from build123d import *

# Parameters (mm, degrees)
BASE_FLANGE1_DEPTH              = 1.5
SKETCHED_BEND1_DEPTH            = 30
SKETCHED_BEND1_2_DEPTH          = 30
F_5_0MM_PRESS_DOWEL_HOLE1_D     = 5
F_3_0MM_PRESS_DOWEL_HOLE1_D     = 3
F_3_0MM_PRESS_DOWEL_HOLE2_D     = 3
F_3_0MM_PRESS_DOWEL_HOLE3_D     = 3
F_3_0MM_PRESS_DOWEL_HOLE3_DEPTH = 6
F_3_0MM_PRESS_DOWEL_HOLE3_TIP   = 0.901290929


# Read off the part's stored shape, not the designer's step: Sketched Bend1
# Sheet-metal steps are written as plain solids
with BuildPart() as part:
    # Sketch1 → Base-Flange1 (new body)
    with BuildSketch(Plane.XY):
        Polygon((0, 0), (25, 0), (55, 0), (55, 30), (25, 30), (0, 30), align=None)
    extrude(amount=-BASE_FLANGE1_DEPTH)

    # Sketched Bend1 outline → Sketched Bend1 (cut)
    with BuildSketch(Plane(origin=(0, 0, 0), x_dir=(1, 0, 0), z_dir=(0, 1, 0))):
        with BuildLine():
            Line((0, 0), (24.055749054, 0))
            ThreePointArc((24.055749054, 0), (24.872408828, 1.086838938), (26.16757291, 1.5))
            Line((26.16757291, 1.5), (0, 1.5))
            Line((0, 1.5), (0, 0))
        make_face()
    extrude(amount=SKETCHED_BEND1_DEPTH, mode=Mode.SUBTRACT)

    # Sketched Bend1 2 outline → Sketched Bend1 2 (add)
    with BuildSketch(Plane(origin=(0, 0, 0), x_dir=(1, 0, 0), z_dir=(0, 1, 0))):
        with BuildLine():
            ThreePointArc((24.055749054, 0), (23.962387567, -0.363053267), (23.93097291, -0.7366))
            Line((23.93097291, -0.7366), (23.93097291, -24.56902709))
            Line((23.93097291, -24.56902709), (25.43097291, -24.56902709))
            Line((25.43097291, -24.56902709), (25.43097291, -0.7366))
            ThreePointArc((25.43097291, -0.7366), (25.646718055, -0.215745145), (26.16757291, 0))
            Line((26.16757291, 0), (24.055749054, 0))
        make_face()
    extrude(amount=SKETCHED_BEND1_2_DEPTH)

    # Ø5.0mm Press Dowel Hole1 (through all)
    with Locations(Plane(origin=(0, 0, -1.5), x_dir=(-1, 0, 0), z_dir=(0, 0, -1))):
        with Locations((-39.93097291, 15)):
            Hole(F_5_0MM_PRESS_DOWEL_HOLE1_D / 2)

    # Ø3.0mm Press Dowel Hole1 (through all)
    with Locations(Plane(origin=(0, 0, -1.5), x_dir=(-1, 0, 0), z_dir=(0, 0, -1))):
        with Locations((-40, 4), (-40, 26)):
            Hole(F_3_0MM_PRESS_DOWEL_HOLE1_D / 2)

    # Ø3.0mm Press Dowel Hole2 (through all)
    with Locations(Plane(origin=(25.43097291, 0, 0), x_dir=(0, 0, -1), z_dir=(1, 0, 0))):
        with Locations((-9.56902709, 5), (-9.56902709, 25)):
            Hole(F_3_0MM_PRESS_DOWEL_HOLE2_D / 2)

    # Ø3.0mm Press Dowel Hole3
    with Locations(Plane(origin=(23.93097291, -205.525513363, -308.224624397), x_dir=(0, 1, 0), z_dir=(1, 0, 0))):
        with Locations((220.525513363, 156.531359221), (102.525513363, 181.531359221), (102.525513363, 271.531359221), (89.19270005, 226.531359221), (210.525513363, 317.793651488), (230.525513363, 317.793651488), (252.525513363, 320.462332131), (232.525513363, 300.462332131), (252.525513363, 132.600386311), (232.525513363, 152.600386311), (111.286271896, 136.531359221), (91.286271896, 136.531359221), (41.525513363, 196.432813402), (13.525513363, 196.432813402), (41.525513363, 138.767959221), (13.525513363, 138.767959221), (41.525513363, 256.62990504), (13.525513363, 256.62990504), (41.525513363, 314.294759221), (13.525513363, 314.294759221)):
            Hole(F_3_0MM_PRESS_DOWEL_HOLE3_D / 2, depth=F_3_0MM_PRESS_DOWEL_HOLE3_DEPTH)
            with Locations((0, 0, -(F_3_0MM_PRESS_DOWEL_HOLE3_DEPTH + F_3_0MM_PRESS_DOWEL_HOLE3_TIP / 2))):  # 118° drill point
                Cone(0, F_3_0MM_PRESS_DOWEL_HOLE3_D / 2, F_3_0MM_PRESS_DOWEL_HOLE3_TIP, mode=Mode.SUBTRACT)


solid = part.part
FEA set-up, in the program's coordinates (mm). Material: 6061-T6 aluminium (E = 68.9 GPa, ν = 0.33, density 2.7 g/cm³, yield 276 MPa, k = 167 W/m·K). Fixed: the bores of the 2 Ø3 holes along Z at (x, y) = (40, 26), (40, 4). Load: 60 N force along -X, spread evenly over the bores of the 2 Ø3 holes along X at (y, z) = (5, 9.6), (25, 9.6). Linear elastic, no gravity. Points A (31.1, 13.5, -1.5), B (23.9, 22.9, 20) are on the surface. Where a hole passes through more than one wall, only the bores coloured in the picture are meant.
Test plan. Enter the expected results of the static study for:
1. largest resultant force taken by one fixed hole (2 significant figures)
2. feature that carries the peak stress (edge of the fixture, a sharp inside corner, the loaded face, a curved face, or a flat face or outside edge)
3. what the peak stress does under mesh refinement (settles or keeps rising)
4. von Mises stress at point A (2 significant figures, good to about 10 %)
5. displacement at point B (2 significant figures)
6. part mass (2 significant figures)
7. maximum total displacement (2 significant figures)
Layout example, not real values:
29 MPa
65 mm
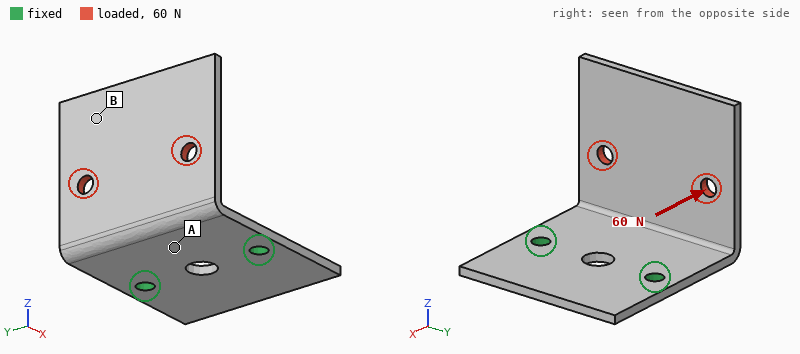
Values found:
31 N
edge of the fixture
keeps rising
45 MPa
0.42 mm
6.5 g
0.51 mm
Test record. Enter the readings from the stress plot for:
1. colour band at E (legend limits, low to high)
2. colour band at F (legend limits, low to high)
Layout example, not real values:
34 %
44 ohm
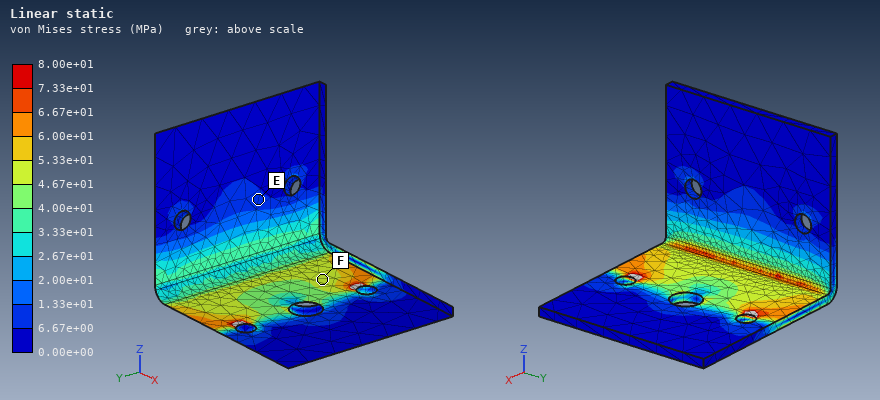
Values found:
6.67e+00 to 1.33e+01 MPa
4.67e+01 to 5.33e+01 MPa
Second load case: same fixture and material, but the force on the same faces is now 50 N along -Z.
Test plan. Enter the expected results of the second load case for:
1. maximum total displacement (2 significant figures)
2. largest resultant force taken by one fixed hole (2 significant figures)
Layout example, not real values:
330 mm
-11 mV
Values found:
0.27 mm
25 N
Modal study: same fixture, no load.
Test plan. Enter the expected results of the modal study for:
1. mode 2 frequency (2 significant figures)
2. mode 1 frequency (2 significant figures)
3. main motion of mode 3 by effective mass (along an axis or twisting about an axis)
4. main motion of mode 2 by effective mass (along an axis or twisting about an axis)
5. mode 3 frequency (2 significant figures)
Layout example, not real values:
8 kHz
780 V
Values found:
2000 Hz
980 Hz
along Z
along Y
3000 Hz
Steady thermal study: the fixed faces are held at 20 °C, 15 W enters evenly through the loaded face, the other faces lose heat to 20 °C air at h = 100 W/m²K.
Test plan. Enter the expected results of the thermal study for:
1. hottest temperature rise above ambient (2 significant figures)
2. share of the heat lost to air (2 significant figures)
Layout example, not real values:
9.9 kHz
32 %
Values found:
40 K
41 %
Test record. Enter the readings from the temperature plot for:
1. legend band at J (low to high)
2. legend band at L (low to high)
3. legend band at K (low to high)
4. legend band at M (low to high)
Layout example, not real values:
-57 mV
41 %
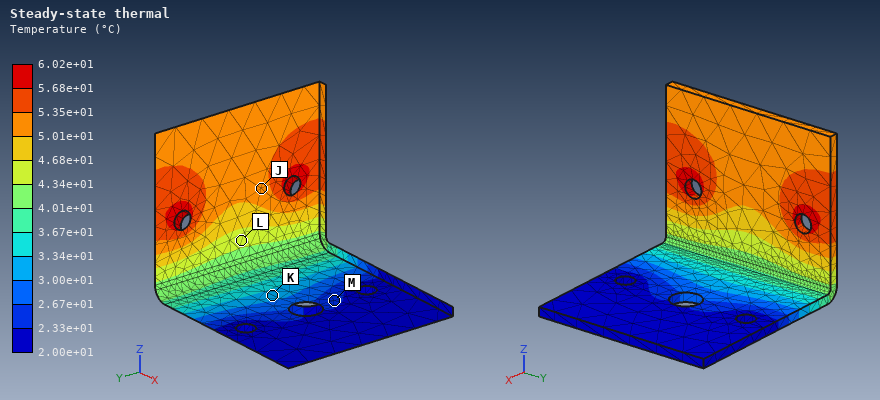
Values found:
5.01e+01 to 5.35e+01 °C
4.34e+01 to 4.68e+01 °C
3.00e+01 to 3.34e+01 °C
2.33e+01 to 2.67e+01 °C
